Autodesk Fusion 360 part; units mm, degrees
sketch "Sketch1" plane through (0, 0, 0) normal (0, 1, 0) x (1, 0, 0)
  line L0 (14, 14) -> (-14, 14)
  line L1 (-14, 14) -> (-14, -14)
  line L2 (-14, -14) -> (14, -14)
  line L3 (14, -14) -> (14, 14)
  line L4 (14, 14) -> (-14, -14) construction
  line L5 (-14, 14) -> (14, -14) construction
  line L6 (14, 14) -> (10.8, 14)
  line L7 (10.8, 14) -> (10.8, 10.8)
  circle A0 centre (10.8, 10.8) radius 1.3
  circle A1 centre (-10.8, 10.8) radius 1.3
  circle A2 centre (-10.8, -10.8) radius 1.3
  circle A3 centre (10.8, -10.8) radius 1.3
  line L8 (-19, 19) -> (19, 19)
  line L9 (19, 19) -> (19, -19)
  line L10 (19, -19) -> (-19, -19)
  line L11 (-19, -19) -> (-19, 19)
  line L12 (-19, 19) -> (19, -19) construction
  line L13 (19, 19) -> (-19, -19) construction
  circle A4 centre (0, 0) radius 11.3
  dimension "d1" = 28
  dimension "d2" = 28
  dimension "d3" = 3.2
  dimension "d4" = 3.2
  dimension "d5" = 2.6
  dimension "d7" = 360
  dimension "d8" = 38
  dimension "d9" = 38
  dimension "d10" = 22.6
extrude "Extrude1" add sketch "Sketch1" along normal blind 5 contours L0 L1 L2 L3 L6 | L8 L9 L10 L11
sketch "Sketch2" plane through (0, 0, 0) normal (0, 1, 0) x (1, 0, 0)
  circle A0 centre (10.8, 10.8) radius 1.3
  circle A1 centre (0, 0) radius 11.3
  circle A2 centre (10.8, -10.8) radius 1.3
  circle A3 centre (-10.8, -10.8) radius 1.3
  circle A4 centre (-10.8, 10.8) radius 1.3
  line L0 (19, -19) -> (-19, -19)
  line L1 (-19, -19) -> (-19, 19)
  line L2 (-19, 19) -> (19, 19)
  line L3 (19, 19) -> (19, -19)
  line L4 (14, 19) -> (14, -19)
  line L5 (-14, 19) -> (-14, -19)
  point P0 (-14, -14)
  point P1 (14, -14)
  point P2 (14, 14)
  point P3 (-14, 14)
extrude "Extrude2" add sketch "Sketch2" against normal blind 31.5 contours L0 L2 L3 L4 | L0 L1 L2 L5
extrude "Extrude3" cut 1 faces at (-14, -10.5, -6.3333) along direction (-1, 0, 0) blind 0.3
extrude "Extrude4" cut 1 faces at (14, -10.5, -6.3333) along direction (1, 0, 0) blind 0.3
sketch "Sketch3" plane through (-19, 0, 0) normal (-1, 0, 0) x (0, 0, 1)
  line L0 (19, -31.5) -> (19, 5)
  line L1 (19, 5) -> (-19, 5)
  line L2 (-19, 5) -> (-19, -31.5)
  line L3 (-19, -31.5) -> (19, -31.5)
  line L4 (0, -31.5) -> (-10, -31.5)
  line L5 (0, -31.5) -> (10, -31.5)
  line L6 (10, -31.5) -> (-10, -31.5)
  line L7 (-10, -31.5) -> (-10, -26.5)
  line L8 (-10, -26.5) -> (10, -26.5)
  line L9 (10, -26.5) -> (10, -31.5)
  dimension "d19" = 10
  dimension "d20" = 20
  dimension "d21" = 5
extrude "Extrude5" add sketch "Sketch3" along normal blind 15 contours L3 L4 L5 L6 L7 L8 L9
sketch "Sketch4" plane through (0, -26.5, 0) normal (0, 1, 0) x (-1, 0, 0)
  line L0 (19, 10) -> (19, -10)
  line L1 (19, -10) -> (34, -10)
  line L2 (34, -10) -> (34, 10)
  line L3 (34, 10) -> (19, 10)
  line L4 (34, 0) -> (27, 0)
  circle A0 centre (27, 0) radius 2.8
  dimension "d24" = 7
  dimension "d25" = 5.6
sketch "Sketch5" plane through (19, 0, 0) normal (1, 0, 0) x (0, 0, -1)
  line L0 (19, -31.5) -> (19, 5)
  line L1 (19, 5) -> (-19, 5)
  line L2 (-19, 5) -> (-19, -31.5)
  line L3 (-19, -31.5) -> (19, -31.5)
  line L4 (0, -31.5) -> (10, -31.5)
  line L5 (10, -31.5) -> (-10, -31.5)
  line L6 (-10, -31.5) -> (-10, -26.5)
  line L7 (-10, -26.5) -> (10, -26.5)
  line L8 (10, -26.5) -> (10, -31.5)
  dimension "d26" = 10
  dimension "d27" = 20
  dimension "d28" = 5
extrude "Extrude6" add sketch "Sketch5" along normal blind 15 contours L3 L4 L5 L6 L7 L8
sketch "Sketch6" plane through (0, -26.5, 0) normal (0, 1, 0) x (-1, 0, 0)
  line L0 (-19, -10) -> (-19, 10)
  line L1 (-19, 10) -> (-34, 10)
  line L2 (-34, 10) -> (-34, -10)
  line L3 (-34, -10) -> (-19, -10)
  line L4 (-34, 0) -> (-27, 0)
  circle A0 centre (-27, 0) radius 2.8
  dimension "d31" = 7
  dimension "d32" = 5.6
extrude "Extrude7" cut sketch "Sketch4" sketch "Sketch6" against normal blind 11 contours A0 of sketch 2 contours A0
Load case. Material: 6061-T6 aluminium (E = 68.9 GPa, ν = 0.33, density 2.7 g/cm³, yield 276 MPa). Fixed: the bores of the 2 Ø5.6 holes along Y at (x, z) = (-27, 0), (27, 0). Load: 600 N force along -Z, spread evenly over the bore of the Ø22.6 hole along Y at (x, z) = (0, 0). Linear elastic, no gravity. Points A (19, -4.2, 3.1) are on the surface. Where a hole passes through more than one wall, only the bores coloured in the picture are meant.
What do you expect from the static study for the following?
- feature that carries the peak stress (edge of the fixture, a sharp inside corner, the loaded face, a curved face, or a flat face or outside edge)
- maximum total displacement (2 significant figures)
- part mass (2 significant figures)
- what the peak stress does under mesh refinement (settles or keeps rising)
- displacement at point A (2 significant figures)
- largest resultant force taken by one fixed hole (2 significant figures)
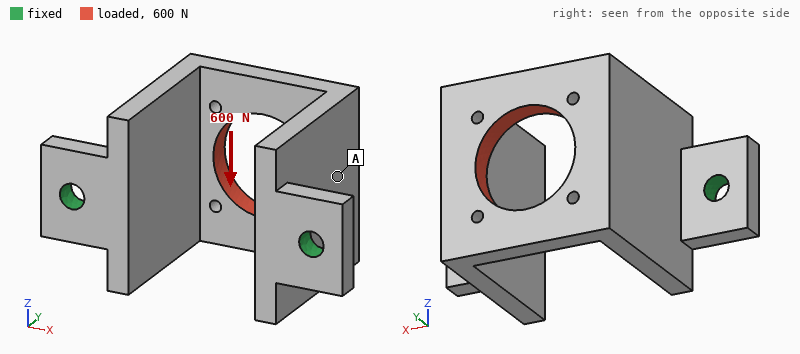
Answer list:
edge of the fixture
0.14 mm
52 g
keeps rising
0.088 mm
300 N
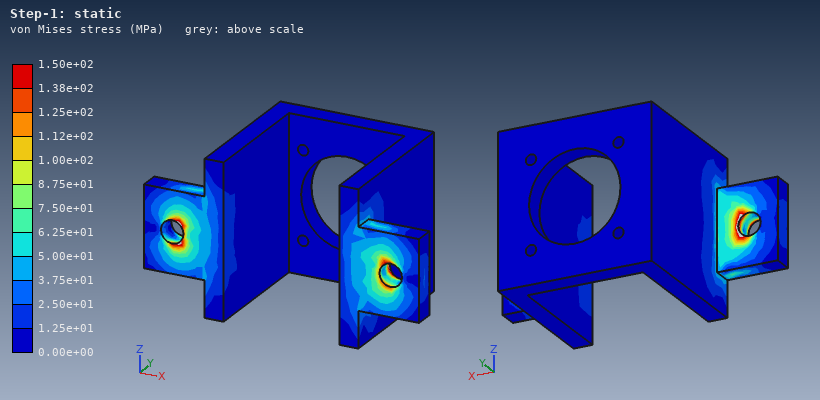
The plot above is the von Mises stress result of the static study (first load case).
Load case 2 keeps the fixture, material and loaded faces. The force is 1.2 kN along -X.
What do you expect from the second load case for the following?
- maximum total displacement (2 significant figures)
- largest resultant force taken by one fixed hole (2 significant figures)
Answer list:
0.17 mm
850 N
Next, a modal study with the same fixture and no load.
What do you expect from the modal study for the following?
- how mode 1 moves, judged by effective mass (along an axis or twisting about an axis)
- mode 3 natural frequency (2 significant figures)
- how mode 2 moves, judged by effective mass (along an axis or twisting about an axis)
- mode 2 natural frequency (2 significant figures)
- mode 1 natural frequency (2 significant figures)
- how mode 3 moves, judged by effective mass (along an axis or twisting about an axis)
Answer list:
along Z
3800 Hz
along X
2900 Hz
2200 Hz
twisting about Y
